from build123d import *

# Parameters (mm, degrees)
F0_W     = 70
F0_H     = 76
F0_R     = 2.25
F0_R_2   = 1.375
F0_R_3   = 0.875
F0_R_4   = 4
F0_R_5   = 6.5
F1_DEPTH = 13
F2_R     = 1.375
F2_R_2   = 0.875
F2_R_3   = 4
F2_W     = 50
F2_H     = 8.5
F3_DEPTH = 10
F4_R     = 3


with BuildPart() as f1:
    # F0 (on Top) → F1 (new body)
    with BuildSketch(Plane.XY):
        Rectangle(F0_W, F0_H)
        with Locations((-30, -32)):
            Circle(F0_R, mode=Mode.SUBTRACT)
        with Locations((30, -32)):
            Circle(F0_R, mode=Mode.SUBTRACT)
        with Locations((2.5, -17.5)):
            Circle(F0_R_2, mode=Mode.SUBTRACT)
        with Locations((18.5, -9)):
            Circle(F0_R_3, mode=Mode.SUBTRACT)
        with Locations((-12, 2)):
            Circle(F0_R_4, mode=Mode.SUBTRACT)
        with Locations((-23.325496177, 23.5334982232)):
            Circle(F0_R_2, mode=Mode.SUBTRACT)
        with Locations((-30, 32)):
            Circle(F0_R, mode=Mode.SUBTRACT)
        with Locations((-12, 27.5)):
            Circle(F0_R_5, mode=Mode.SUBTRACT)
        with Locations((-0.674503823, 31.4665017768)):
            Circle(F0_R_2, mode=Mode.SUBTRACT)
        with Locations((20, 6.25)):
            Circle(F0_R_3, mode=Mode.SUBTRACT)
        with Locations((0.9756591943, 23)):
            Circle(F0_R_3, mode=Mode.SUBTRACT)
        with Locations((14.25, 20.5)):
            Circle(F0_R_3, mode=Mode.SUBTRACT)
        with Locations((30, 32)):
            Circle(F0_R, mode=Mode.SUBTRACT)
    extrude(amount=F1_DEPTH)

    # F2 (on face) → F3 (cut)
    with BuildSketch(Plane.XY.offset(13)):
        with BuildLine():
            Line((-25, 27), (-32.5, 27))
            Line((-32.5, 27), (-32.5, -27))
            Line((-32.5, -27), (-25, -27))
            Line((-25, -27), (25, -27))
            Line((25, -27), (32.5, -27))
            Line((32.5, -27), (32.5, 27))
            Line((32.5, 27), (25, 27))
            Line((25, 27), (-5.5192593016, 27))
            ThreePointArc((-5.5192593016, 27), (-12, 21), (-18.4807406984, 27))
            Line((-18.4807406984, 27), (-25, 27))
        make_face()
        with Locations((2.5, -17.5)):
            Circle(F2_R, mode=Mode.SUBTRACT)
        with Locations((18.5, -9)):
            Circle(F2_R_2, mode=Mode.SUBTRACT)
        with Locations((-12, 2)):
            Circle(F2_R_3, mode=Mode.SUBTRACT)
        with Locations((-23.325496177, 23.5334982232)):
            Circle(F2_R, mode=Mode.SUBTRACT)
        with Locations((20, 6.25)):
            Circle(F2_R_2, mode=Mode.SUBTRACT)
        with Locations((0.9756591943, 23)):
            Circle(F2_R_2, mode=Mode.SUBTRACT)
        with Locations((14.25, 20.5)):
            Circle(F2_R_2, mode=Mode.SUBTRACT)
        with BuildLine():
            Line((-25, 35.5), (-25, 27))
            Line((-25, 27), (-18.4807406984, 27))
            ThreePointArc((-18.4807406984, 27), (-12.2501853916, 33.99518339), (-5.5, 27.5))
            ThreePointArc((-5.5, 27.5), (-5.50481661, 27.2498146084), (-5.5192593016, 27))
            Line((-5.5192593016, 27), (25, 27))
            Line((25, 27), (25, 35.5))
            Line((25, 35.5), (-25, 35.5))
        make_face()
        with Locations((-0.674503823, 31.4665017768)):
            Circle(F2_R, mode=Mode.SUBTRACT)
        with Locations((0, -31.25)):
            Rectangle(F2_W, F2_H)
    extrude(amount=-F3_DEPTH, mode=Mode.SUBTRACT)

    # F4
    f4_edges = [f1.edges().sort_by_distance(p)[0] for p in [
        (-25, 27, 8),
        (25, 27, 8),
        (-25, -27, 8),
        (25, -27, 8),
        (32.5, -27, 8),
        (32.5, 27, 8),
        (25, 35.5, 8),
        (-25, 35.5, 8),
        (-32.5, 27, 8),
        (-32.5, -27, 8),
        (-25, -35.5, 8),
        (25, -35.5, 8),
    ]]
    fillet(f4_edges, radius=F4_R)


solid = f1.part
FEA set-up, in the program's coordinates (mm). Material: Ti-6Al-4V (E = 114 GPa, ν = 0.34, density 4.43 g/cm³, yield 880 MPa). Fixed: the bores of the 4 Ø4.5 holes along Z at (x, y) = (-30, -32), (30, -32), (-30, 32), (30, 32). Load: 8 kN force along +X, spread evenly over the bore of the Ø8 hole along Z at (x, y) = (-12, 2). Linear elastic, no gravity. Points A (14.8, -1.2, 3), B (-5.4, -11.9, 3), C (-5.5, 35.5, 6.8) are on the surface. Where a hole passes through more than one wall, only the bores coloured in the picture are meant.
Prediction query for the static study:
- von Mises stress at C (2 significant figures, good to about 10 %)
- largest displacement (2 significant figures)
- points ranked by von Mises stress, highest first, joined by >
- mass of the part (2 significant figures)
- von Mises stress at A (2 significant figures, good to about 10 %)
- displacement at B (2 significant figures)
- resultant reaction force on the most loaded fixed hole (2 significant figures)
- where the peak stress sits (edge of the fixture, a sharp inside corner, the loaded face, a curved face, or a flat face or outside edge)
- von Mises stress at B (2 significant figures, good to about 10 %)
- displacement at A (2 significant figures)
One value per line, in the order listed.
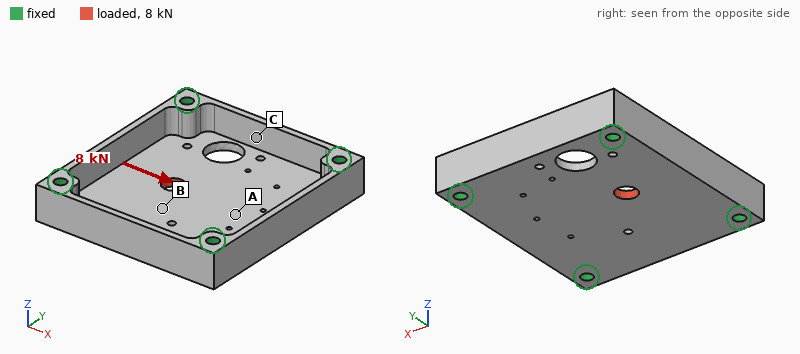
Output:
12 MPa
28 µm
B > A > C
110 g
25 MPa
14 µm
2.3 kN
the loaded face
44 MPa
14 µm
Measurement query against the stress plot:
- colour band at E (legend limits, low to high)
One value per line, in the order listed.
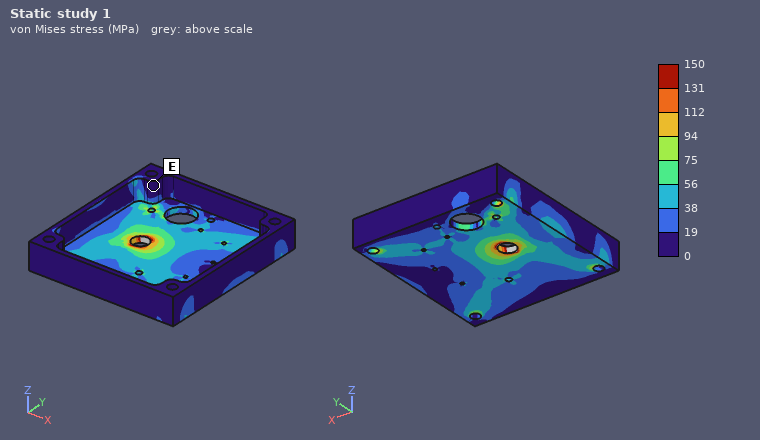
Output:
0 to 19 MPa
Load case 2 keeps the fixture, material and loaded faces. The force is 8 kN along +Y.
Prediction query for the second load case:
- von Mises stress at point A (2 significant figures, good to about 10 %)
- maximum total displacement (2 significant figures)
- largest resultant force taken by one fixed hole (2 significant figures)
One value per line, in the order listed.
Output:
18 MPa
22 µm
2.8 kN
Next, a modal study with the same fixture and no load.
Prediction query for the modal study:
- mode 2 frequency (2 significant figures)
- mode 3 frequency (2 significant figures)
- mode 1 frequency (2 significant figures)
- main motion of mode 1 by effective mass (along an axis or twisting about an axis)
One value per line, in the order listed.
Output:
7800 Hz
8100 Hz
3800 Hz
along Z
